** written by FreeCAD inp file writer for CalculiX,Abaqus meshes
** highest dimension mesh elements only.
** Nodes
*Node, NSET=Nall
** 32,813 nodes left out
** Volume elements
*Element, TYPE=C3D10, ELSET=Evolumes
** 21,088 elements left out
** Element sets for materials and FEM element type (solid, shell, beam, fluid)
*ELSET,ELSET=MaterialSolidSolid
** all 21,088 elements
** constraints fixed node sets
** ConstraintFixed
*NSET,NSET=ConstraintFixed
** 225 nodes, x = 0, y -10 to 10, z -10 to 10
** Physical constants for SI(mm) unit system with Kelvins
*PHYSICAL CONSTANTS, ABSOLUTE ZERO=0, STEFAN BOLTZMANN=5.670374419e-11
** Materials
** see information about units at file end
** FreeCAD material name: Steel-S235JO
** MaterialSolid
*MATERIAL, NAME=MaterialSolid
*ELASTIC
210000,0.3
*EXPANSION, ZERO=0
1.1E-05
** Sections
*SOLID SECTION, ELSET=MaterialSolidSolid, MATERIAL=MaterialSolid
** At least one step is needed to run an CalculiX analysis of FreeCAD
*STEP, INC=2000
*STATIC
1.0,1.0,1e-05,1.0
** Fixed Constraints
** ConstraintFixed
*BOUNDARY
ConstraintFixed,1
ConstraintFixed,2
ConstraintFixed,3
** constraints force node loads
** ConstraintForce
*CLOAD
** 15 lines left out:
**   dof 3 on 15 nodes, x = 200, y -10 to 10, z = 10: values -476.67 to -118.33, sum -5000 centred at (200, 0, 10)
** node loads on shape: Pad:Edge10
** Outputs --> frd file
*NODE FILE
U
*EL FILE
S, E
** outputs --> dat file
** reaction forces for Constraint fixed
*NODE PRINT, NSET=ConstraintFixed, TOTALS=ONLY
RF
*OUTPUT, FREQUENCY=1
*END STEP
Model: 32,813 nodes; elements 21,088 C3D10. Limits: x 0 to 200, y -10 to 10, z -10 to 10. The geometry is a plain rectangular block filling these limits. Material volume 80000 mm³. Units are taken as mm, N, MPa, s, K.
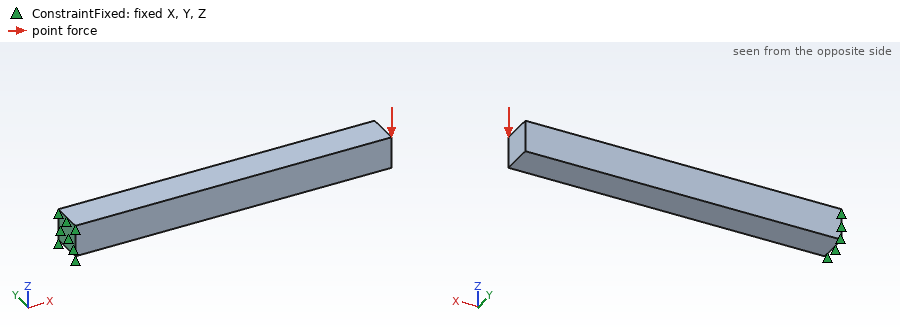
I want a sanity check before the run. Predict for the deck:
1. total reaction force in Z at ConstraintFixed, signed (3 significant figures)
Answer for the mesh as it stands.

5000 N
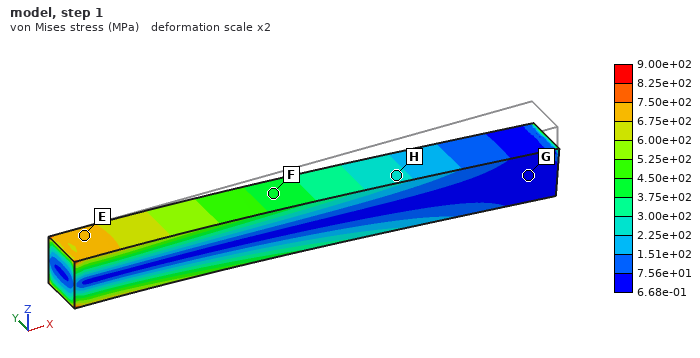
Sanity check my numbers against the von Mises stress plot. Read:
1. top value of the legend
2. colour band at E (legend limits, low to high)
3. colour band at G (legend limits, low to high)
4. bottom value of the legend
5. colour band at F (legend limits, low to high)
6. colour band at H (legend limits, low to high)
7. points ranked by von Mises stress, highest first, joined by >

9.00e+02 MPa
6.75e+02 to 7.50e+02 MPa
6.68e-01 to 7.56e+01 MPa
6.68e-01 MPa
3.75e+02 to 4.50e+02 MPa
2.25e+02 to 3.00e+02 MPa
E > F > H > G
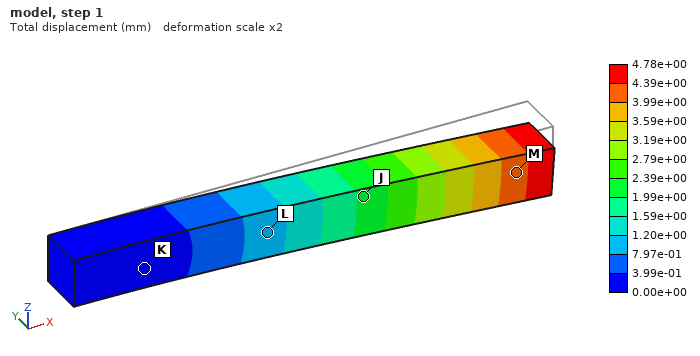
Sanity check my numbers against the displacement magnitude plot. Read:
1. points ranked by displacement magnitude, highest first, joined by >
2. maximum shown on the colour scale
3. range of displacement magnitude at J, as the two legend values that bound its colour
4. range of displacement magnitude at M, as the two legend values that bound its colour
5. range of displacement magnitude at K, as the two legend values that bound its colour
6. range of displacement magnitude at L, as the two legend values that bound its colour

M > J > L > K
4.78e+00 mm
1.99e+00 to 2.39e+00 mm
3.99e+00 to 4.39e+00 mm
0.00e+00 to 3.99e-01 mm
7.97e-01 to 1.20e+00 mm
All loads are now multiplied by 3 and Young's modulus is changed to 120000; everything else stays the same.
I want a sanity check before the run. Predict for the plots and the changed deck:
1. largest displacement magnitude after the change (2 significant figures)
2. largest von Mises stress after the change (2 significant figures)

25 mm
2700 MPa
